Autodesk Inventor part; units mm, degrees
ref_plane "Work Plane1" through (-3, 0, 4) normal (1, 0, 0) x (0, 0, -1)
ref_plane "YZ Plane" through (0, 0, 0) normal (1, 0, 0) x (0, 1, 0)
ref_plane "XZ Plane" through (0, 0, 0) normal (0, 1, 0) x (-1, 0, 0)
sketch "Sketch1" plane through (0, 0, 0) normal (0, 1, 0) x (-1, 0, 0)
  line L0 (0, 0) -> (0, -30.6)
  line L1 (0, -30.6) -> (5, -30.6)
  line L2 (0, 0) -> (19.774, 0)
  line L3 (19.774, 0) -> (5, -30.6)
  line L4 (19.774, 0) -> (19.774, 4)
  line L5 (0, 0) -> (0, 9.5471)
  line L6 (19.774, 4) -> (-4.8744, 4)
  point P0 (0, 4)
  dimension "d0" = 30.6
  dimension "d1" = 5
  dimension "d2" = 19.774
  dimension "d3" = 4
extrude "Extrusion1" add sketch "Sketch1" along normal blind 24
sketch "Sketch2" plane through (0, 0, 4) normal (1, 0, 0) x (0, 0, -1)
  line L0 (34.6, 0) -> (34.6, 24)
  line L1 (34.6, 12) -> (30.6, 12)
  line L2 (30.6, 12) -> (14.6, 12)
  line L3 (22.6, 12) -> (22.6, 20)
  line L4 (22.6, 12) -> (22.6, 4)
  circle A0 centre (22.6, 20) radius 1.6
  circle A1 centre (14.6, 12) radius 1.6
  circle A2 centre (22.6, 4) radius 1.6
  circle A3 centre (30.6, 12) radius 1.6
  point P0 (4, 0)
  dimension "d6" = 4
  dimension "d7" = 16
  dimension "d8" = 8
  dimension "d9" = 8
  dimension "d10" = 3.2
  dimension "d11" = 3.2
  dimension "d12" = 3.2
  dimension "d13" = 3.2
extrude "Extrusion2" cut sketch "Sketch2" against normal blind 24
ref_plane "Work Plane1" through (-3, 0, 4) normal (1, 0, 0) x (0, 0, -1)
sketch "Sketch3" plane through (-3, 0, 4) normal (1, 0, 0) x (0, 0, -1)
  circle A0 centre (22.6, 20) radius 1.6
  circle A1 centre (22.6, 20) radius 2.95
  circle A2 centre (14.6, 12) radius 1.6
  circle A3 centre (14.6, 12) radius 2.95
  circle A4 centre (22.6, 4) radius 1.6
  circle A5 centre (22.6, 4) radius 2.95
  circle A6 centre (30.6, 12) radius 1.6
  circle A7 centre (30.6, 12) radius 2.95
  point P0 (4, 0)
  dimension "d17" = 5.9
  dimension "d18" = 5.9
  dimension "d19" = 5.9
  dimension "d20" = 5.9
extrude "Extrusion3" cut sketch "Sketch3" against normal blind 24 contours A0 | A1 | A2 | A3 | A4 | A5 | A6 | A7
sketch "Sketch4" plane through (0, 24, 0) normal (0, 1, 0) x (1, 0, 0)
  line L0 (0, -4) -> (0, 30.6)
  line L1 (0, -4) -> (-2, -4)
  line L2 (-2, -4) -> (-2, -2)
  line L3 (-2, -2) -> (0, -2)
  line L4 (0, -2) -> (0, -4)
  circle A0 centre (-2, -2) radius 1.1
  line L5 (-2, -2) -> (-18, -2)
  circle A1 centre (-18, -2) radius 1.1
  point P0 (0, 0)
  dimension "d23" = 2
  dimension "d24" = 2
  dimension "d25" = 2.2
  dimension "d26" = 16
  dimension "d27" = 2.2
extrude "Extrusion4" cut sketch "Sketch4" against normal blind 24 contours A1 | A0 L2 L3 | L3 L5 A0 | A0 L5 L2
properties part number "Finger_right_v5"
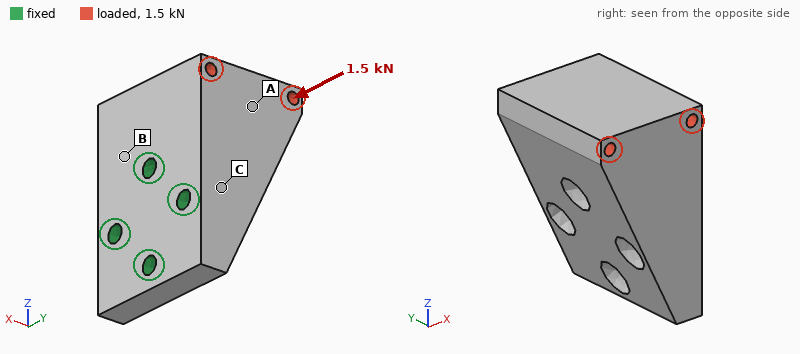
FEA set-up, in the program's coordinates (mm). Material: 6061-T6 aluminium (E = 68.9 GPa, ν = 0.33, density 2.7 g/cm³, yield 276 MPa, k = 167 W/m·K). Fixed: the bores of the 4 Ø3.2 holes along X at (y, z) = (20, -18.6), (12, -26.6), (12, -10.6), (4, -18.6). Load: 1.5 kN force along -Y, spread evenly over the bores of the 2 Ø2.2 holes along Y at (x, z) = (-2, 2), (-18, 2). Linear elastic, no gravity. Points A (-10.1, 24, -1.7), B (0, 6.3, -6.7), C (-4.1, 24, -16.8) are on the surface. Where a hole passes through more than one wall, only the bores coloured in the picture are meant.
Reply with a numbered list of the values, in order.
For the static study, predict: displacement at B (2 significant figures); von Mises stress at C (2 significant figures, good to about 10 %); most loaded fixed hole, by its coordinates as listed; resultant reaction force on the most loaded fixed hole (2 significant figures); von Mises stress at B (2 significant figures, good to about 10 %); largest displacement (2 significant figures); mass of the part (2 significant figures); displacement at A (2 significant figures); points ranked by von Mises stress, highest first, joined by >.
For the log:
1. 4.7 µm
2. 27 MPa
3. (12, -10.6)
4. 1.4 kN
5. 15 MPa
6. 22 µm
7. 27 g
8. 14 µm
9. C > B > A
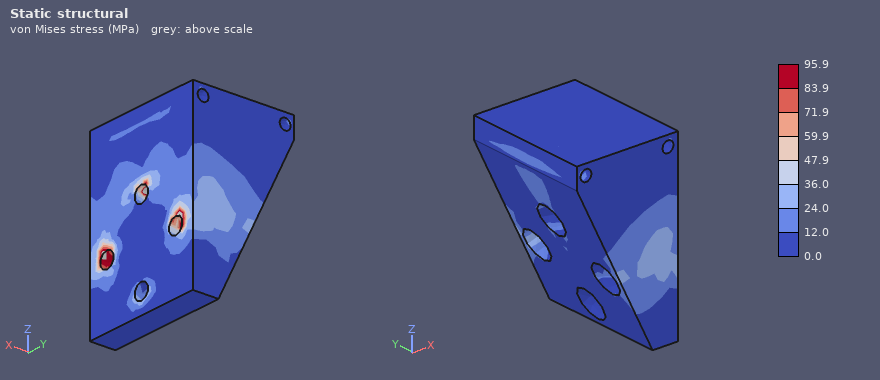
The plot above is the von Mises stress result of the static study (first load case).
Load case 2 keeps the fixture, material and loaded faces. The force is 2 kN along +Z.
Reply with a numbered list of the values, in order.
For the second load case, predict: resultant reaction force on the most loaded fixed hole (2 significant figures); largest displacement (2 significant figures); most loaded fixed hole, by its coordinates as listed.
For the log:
1. 1.2 kN
2. 25 µm
3. (12, -10.6)
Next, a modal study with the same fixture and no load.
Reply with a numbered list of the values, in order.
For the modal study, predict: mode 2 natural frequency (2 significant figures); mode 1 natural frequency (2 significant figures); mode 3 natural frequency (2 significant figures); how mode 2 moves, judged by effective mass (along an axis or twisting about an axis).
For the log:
1. 14 kHz
2. 10 kHz
3. 21 kHz
4. along Y
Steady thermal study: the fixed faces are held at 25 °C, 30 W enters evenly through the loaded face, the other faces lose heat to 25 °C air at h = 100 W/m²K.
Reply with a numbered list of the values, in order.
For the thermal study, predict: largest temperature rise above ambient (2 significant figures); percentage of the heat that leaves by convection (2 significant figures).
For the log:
1. 14 K
2. 7.7 %
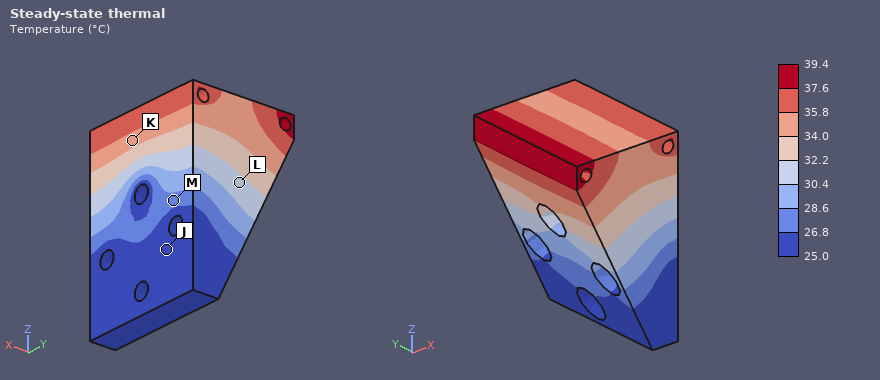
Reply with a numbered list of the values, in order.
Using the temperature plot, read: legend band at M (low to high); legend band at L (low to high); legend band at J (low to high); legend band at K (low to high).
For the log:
1. 26.8 to 28.6 °C
2. 30.4 to 32.2 °C
3. 25.0 to 26.8 °C
4. 34.0 to 35.8 °C
